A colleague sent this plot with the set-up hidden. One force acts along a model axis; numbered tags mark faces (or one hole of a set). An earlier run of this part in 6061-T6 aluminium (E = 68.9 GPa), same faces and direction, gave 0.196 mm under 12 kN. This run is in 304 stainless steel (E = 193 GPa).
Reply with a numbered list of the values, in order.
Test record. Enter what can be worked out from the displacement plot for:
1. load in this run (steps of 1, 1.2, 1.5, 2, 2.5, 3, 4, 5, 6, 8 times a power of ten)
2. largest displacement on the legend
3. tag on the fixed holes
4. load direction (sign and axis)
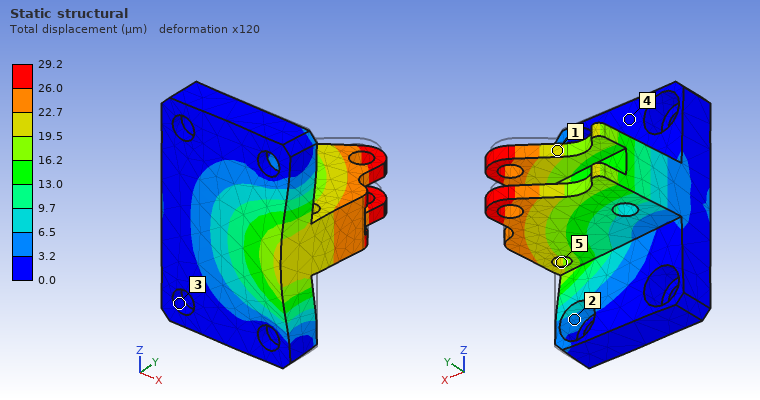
1. 5 kN
2. 29.2 µm
3. 3
4. -Y
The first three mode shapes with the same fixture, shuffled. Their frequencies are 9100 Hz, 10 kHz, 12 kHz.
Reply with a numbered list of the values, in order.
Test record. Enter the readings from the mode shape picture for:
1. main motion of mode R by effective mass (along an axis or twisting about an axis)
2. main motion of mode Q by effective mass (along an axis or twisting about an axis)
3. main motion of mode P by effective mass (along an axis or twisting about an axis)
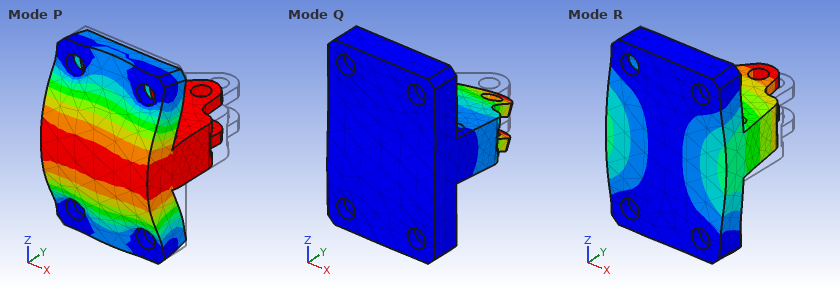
1. along X
2. along Z
3. along Y
